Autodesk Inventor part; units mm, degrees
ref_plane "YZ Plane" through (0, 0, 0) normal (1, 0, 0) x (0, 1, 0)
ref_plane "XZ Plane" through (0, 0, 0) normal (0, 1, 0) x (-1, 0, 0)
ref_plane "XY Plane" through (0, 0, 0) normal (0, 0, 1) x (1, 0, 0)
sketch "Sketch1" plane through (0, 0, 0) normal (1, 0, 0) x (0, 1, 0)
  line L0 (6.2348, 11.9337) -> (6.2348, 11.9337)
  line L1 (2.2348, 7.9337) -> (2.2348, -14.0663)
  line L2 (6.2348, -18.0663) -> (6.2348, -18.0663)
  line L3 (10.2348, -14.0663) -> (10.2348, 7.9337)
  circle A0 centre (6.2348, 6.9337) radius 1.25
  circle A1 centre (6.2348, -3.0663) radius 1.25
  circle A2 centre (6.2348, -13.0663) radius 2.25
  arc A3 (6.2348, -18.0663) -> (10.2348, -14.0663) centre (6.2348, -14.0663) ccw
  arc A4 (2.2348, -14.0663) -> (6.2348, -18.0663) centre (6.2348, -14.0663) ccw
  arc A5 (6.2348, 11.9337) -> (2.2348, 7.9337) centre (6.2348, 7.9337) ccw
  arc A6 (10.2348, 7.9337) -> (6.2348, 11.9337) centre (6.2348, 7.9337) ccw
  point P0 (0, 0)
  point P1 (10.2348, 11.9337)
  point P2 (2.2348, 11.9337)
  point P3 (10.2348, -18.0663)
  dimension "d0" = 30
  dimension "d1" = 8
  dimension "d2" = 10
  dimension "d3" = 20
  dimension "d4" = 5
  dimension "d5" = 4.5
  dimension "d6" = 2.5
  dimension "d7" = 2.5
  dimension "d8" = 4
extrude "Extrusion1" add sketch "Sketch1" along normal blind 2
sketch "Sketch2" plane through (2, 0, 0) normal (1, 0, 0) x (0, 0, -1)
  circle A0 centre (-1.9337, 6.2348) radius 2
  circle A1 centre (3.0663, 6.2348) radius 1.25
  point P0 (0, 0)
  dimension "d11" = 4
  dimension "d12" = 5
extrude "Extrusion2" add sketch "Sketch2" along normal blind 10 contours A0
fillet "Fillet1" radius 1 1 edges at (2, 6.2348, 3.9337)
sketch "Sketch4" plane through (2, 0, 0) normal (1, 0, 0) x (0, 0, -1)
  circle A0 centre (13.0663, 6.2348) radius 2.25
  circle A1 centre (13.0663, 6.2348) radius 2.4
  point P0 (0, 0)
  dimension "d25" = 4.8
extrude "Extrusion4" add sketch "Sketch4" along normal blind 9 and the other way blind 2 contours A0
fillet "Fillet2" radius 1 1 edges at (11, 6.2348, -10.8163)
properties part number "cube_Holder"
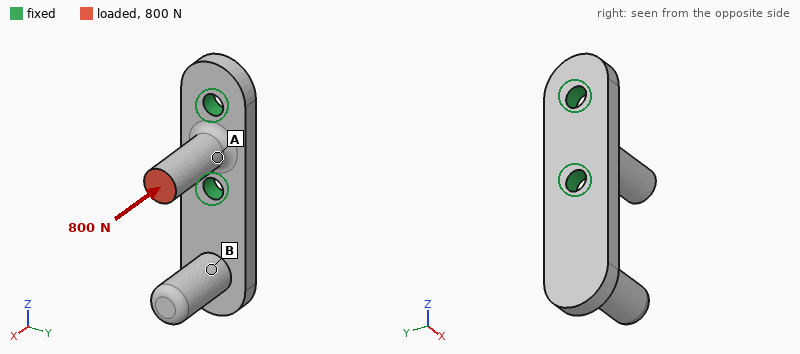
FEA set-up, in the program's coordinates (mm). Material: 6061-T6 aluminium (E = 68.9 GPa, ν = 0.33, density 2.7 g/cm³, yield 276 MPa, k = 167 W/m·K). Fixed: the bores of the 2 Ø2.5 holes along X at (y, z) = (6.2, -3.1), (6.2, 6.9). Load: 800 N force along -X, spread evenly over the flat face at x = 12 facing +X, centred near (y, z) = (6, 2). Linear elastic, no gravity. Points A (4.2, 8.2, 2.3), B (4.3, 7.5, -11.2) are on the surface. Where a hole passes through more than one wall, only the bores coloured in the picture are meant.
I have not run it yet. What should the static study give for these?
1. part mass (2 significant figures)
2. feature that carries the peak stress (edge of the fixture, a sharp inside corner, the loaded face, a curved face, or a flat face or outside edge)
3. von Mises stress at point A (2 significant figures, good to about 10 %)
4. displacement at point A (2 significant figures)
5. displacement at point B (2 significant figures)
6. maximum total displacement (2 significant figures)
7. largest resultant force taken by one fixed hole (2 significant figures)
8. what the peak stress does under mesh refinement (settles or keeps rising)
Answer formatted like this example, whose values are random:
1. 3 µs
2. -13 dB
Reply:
1. 1.9 g
2. edge of the fixture
3. 58 MPa
4. 9.2 µm
5. 2.9 µm
6. 16 µm
7. 420 N
8. keeps rising
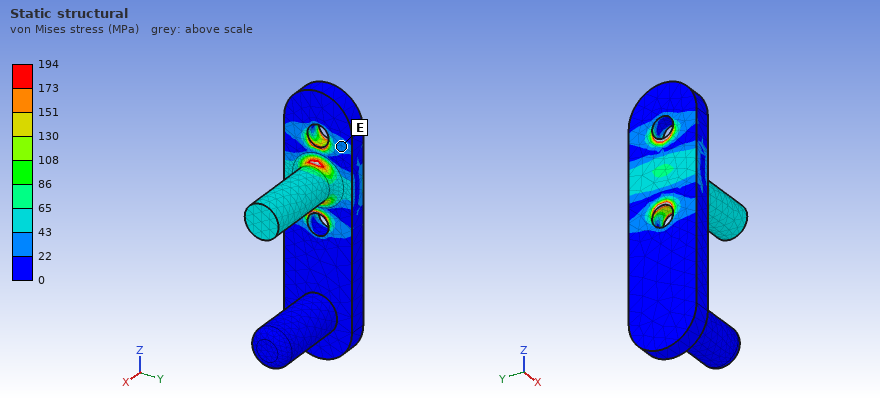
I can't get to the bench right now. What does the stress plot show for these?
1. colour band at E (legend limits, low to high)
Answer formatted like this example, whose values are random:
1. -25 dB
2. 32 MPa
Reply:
1. 22 to 43 MPa
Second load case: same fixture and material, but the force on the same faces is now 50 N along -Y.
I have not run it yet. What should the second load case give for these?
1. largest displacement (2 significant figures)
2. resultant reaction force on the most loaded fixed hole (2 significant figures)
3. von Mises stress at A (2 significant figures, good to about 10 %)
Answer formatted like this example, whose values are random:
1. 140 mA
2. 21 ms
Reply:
1. 37 µm
2. 25 N
3. 60 MPa
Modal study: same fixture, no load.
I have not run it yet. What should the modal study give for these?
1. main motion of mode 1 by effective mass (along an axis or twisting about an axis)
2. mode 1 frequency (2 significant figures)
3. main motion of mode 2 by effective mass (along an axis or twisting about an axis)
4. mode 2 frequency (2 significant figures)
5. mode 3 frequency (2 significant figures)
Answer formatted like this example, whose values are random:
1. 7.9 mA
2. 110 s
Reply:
1. along X
2. 5300 Hz
3. along Y
4. 9100 Hz
5. 18 kHz
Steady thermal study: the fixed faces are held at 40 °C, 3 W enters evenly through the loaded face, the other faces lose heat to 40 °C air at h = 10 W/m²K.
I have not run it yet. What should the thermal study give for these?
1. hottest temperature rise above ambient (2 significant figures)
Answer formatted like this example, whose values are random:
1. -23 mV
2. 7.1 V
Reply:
1. 17 K
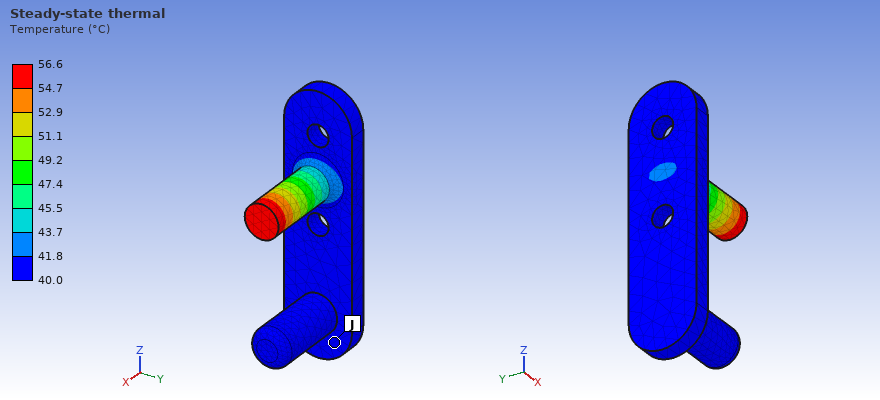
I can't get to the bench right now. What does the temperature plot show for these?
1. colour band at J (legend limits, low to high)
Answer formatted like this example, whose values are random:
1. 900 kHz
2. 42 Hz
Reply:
1. 40.0 to 41.8 °C
